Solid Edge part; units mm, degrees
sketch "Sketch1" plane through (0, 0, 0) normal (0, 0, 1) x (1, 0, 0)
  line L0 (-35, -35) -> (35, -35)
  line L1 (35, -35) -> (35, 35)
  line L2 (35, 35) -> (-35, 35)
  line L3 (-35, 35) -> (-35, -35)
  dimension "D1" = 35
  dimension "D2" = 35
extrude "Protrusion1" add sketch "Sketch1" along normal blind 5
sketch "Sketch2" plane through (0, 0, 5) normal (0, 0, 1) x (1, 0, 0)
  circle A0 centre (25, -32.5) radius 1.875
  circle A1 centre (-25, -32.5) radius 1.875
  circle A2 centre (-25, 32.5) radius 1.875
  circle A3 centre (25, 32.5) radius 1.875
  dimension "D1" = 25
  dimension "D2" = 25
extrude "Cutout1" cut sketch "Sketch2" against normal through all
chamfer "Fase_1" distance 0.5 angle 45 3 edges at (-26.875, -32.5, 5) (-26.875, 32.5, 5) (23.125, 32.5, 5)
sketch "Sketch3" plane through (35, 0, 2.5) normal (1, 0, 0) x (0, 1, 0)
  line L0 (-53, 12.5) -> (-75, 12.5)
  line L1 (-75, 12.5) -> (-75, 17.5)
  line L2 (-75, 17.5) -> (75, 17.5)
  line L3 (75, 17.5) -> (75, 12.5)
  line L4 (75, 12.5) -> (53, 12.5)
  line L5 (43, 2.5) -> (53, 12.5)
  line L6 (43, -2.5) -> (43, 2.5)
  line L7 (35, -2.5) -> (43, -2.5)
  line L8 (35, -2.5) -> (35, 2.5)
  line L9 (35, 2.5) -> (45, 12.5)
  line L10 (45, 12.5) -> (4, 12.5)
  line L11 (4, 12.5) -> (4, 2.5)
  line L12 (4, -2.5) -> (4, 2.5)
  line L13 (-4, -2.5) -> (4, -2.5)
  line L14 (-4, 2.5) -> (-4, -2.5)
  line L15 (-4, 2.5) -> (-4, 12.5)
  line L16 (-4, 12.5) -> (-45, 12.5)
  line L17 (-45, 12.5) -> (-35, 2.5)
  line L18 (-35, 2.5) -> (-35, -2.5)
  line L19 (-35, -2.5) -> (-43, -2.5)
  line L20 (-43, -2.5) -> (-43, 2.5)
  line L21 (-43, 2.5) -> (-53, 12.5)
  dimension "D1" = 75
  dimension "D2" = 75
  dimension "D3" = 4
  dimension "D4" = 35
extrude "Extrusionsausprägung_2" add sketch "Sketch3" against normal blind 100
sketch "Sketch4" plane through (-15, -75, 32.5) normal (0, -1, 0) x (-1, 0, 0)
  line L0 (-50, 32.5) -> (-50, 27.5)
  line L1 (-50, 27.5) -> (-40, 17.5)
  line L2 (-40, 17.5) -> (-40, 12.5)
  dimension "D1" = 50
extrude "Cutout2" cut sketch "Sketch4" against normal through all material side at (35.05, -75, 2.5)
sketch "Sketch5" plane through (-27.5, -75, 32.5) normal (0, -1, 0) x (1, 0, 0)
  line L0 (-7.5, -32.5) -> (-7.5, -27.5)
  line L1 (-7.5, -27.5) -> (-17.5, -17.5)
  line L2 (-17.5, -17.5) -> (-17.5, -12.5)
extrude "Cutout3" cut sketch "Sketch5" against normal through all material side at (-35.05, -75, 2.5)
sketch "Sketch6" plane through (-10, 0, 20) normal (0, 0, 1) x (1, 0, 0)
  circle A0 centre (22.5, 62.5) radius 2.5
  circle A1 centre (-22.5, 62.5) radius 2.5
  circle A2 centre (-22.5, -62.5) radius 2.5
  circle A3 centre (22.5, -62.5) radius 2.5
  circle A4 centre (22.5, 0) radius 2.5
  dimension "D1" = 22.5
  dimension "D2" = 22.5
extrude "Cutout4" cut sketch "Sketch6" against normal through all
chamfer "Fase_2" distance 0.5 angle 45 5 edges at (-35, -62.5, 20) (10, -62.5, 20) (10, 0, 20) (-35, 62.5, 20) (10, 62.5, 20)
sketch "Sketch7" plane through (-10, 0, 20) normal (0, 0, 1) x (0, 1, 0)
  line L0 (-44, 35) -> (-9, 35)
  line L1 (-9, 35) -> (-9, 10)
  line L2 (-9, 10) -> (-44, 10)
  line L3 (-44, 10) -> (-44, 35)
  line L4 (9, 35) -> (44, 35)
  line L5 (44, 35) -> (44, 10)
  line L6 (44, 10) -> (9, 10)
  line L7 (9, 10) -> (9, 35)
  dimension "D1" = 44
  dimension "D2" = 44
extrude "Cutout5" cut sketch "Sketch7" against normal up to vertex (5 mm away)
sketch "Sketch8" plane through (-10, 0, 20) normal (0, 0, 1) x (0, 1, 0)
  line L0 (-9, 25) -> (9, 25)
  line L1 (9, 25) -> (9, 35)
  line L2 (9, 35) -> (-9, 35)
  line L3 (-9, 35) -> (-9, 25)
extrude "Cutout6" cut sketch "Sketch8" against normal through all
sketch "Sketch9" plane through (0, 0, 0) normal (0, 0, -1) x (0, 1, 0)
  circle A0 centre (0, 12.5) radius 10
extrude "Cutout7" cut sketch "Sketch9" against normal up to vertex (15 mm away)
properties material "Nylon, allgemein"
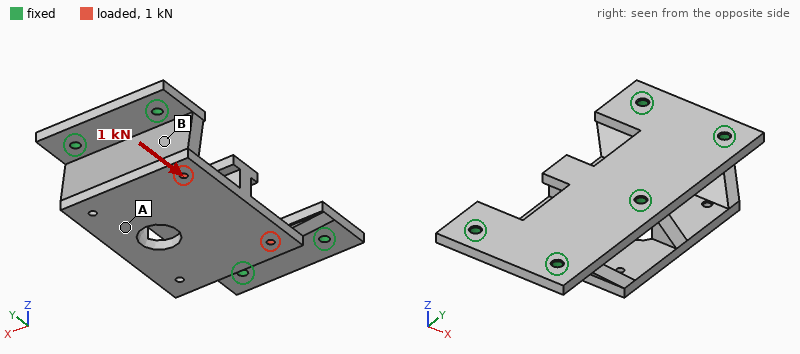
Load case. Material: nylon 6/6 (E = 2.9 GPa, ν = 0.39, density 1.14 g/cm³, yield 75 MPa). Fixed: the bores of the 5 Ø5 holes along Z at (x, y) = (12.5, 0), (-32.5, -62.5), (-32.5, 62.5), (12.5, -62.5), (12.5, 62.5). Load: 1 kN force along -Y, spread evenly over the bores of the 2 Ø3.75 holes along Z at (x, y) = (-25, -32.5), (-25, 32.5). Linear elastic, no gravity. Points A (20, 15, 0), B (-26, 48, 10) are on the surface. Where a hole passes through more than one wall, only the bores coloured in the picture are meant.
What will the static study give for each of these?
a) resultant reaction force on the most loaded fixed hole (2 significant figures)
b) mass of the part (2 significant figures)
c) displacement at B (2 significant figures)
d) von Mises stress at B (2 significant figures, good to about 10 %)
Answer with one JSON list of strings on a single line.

["320 N", "97 g", "0.085 mm", "3.5 MPa"]
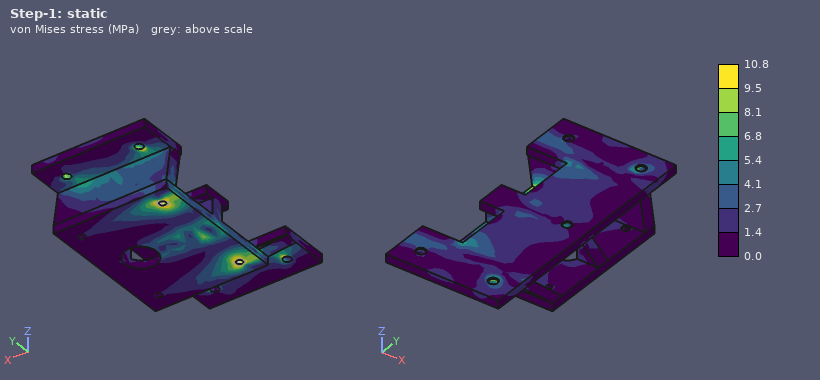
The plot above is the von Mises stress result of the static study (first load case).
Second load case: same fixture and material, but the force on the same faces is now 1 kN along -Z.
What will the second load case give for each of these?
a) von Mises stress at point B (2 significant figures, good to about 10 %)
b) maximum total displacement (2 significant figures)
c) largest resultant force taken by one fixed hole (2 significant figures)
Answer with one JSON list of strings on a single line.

["8.5 MPa", "0.37 mm", "610 N"]
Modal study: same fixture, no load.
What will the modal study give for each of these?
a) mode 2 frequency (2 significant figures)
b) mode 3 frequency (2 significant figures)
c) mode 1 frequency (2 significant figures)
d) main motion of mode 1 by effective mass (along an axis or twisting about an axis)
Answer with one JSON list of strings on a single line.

["1800 Hz", "1800 Hz", "1400 Hz", "along Z"]
